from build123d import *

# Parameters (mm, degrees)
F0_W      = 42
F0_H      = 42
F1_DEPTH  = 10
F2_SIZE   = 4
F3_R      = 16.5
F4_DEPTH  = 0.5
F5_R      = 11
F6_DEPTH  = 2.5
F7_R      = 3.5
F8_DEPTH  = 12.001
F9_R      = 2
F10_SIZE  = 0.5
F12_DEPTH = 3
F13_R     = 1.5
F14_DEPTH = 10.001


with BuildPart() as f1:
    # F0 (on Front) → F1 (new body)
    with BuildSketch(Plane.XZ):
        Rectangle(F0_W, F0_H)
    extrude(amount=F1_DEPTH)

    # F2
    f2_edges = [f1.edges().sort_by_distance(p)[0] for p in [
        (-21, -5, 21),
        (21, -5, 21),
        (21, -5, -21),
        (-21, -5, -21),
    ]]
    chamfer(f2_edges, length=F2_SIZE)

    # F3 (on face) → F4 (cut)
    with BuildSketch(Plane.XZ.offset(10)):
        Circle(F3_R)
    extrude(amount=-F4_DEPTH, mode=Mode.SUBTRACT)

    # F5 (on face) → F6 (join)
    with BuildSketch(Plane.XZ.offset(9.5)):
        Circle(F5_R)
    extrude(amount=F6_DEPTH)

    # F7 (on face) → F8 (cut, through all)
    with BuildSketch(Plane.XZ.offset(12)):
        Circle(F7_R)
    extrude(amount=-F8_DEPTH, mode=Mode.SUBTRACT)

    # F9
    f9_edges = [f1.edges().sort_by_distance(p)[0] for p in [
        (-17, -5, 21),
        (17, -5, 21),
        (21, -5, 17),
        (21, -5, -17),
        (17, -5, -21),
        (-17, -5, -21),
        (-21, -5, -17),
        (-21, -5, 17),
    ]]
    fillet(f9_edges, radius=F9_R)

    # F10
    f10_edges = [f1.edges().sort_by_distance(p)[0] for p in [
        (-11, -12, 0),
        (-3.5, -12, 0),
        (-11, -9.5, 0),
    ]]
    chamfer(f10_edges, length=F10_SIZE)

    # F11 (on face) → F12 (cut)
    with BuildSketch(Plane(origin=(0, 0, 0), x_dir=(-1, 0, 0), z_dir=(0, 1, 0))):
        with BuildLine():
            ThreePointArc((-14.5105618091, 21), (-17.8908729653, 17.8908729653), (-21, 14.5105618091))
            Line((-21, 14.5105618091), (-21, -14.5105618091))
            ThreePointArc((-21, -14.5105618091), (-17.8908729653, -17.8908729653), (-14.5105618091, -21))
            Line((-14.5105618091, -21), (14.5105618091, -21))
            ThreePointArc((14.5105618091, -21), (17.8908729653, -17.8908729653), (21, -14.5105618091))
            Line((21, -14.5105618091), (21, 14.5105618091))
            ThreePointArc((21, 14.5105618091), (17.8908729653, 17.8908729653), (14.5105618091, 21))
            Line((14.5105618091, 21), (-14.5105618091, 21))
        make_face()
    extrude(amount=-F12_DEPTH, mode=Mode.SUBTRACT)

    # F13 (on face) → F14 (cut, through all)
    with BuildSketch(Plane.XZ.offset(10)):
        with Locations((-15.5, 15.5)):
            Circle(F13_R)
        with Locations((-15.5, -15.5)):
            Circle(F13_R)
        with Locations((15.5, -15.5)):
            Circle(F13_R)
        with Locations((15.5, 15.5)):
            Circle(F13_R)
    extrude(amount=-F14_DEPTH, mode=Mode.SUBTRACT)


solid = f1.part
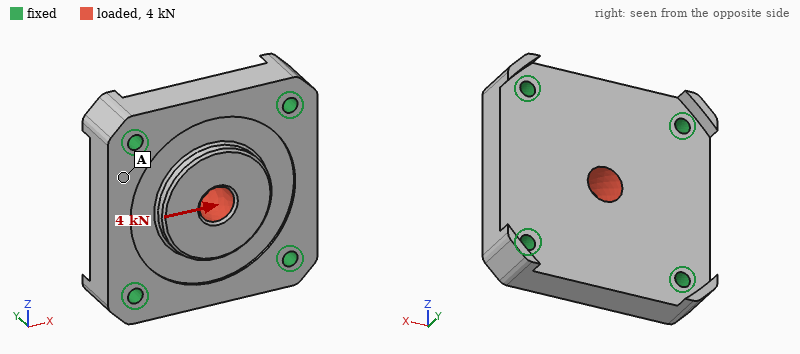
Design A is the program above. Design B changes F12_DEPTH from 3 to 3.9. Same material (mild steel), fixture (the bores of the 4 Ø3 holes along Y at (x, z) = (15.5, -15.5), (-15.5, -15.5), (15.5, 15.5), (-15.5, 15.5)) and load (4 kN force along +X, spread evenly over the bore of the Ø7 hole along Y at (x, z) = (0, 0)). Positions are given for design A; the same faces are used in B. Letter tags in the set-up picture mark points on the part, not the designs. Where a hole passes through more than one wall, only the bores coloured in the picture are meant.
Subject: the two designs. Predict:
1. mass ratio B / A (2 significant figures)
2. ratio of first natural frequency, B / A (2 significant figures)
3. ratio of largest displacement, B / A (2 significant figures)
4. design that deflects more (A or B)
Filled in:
0.88
0.92
1.1
B
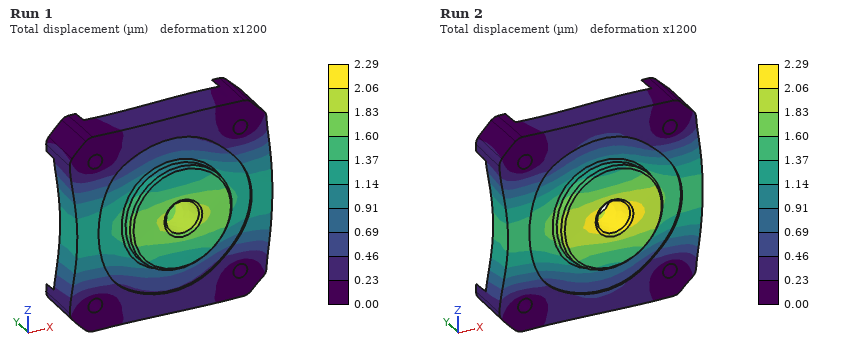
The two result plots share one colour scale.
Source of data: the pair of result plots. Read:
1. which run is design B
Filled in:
Run 2
